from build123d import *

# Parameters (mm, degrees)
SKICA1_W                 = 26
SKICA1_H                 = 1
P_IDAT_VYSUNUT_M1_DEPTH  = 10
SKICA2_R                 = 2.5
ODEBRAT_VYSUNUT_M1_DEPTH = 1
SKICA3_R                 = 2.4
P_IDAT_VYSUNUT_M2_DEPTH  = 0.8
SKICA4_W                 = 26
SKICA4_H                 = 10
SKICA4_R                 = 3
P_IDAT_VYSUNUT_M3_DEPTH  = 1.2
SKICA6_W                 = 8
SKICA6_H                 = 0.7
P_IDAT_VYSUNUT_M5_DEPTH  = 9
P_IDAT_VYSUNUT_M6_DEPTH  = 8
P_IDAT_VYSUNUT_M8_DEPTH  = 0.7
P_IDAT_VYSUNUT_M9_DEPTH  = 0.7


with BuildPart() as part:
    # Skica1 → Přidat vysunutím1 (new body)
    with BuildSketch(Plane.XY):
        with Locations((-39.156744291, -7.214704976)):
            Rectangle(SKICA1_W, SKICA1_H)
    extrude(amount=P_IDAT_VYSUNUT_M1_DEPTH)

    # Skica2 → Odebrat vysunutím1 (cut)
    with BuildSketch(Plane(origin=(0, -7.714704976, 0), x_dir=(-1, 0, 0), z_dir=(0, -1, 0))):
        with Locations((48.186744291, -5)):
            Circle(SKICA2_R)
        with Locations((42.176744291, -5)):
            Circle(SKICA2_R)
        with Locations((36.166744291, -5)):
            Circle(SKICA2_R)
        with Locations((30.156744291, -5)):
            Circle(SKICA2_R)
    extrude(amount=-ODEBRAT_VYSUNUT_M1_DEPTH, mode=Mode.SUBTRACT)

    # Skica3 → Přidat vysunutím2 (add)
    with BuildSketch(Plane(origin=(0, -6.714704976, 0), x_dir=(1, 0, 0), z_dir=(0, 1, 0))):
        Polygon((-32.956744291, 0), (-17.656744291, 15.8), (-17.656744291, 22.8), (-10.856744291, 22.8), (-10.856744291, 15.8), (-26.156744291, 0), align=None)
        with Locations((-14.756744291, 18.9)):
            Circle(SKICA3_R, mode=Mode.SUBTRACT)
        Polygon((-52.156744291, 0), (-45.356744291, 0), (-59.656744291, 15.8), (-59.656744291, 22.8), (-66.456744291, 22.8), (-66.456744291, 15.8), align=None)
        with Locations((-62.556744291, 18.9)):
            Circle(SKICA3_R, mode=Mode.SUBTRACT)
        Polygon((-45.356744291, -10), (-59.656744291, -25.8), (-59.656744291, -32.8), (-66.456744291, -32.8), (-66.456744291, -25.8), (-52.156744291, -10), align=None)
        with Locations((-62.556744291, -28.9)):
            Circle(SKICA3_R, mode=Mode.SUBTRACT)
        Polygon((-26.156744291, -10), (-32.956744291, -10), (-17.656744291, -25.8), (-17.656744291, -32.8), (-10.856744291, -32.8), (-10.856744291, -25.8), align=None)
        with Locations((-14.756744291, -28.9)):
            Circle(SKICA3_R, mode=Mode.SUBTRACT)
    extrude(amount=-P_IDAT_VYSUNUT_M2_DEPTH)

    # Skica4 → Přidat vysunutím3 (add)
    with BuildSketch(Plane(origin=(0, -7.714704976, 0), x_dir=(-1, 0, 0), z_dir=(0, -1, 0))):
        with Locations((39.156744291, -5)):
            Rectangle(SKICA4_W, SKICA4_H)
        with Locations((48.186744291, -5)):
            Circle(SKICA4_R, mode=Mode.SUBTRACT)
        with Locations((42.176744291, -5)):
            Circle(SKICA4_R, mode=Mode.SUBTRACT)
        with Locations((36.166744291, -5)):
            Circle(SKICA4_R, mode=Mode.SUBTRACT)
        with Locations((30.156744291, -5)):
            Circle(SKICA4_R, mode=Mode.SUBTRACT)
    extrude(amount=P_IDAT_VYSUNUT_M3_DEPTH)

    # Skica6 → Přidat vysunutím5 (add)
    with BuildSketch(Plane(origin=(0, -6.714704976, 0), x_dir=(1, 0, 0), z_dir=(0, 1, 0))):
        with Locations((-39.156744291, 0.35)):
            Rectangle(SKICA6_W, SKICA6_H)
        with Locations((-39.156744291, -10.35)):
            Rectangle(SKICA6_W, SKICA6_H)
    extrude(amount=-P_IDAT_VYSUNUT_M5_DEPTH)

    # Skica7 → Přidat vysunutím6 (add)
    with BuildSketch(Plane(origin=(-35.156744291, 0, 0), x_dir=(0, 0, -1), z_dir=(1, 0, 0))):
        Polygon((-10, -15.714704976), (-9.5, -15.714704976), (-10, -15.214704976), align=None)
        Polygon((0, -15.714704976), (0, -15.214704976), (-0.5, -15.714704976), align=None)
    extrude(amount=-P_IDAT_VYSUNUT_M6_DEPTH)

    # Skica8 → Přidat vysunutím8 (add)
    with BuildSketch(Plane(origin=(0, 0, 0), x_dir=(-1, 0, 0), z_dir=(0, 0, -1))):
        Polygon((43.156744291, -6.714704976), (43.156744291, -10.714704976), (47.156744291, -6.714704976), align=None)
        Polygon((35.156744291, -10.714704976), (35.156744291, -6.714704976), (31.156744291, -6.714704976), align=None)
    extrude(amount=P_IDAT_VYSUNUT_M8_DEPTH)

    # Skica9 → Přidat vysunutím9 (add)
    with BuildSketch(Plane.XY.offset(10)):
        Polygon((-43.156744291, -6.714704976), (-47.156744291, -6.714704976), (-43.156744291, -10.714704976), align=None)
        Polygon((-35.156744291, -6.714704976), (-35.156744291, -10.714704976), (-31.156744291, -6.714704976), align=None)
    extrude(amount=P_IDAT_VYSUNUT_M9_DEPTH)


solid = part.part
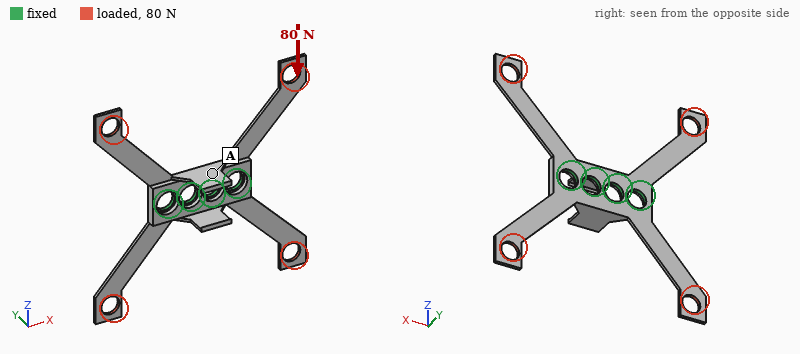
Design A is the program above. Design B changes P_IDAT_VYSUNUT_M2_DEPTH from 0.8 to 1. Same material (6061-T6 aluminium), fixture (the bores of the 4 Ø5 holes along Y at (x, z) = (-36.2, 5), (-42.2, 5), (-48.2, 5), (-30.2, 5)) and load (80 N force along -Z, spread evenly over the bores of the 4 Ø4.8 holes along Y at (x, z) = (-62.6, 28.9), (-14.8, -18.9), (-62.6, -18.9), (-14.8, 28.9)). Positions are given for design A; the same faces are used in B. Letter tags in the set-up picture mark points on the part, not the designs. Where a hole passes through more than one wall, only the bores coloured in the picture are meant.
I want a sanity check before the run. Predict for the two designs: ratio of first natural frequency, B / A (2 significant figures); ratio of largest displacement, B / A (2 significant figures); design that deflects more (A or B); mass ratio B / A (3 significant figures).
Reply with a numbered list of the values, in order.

1. 1.2
2. 0.80
3. A
4. 1.12
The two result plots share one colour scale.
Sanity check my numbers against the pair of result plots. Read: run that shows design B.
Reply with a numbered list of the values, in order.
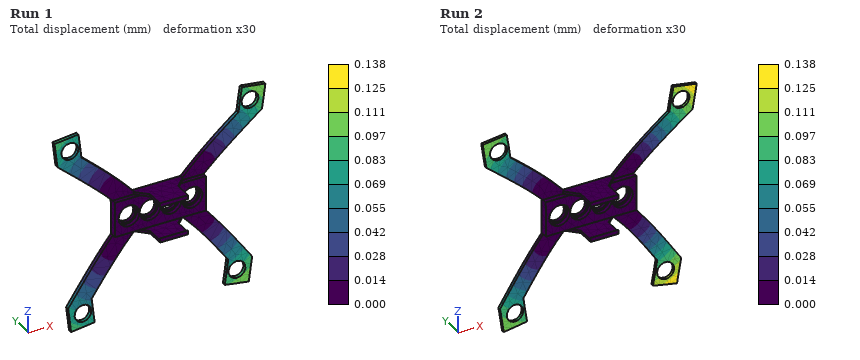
1. Run 1
